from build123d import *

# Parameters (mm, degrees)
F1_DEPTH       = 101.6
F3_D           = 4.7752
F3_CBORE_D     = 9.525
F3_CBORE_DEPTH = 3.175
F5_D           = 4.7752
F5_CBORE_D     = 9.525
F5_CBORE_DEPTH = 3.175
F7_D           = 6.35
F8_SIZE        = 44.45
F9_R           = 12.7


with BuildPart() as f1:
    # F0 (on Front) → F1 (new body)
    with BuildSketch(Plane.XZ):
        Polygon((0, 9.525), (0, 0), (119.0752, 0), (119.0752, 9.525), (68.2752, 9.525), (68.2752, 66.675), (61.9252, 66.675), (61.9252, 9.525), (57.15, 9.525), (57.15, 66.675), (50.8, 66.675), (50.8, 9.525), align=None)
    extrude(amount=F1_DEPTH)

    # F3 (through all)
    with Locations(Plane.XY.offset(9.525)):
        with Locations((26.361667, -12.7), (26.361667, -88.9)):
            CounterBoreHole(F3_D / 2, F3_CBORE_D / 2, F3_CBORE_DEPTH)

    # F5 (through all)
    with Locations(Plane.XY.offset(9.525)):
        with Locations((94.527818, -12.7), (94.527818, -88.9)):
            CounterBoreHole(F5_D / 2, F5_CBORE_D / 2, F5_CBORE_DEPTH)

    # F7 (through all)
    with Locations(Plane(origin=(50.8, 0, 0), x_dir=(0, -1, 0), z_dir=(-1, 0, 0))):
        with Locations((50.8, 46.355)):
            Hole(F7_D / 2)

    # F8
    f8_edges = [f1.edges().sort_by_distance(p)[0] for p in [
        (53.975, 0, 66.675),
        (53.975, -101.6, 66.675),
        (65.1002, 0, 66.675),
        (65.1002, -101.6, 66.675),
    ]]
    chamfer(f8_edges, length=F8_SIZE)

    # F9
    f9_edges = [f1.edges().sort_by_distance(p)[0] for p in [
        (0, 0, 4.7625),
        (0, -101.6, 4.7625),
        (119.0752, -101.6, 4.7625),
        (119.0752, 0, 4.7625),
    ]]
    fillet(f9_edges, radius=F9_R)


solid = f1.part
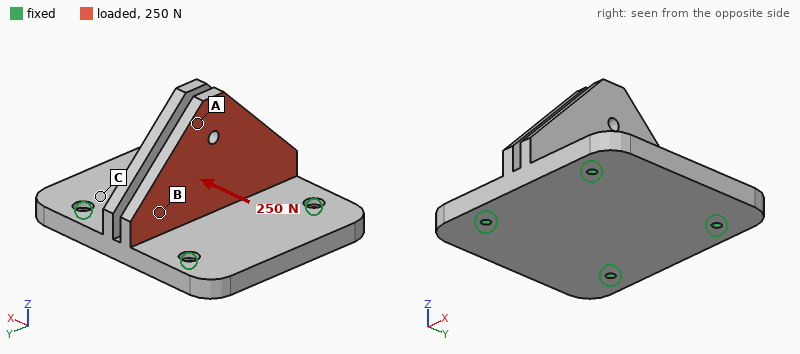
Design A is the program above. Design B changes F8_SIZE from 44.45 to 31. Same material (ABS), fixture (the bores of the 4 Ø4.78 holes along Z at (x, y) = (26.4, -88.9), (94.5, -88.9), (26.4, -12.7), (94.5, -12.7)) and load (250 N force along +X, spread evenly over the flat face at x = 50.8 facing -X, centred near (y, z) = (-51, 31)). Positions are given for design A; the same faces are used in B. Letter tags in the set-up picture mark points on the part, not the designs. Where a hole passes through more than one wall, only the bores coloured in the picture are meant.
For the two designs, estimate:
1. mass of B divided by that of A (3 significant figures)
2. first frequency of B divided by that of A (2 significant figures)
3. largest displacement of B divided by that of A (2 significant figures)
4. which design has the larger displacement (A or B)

1.08
0.82
1.1
B
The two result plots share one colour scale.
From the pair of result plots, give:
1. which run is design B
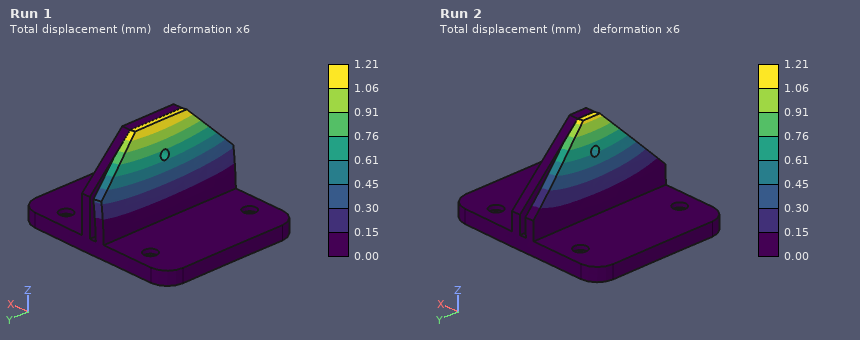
Run 1
